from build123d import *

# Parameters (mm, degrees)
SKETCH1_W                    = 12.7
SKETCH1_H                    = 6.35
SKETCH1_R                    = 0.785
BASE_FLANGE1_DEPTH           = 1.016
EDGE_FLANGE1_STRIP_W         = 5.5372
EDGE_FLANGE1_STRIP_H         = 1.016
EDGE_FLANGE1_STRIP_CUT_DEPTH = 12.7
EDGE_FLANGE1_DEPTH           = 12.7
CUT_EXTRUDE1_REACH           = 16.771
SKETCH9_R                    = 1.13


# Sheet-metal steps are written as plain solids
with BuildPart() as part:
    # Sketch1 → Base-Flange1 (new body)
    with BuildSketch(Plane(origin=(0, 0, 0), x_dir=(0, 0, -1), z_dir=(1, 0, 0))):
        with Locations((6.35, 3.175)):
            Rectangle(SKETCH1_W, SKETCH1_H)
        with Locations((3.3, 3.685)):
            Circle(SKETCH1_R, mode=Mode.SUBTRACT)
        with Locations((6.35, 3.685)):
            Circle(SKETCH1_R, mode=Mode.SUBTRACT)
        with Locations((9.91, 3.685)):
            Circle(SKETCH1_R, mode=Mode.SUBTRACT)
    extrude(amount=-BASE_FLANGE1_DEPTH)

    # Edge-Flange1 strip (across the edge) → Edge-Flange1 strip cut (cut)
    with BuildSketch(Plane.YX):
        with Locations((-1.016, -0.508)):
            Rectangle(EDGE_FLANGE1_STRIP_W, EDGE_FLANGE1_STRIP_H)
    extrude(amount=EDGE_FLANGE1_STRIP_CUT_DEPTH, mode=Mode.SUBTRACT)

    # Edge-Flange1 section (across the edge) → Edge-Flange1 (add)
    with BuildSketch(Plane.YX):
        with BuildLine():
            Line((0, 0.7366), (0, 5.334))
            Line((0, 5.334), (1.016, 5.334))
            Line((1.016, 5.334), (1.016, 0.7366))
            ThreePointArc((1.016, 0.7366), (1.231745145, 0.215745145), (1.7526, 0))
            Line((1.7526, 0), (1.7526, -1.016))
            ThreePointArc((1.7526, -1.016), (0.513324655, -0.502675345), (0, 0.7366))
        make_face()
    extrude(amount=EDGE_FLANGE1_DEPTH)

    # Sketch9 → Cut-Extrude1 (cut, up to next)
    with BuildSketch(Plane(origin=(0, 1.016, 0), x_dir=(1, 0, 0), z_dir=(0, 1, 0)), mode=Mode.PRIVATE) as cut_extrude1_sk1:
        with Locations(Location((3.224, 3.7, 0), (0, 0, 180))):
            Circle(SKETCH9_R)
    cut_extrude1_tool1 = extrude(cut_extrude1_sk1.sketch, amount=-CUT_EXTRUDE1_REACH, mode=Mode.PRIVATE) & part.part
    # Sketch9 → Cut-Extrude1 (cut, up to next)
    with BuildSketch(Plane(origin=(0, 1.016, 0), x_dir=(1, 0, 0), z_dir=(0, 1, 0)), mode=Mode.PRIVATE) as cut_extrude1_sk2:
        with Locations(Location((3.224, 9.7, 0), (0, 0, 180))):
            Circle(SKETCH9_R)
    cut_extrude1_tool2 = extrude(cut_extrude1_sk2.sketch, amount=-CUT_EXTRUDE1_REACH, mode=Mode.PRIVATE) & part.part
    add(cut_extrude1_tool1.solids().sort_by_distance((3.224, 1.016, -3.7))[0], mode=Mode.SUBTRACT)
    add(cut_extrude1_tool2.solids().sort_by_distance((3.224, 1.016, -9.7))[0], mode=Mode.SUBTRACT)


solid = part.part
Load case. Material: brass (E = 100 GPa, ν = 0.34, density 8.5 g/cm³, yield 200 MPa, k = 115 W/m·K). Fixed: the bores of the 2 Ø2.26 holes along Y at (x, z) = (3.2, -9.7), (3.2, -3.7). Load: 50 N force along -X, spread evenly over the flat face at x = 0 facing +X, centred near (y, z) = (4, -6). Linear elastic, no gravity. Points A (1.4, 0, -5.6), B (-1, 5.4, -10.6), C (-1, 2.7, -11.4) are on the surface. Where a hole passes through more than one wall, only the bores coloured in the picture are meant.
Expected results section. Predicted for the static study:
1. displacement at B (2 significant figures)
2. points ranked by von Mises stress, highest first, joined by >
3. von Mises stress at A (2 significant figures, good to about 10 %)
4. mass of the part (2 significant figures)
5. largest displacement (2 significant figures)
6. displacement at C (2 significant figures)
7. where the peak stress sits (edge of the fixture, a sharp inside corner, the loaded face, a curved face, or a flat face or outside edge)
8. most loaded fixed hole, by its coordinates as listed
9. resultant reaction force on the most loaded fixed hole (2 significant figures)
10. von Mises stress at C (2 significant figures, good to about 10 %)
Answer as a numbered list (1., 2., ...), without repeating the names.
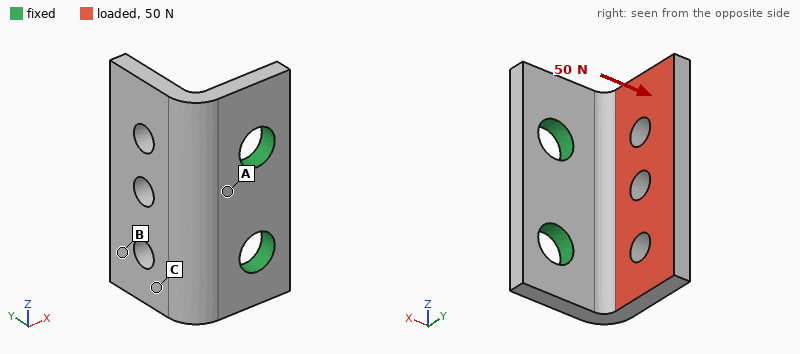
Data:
1. 31 µm
2. A > C > B
3. 66 MPa
4. 1.1 g
5. 38 µm
6. 15 µm
7. a flat face or outside edge
8. (3.2, -3.7)
9. 27 N
10. 39 MPa
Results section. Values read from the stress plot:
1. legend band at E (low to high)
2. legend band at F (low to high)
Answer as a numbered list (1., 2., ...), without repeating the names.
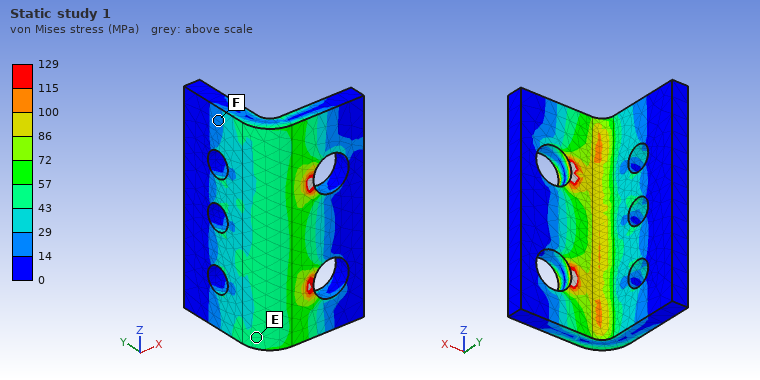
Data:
1. 43 to 57 MPa
2. 14 to 29 MPa
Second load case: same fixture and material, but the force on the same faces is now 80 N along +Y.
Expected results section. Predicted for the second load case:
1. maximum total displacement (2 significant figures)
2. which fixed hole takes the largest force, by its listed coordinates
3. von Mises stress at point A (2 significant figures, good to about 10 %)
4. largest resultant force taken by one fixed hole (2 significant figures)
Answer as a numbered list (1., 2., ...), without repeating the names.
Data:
1. 12 µm
2. (3.2, -3.7)
3. 39 MPa
4. 44 N
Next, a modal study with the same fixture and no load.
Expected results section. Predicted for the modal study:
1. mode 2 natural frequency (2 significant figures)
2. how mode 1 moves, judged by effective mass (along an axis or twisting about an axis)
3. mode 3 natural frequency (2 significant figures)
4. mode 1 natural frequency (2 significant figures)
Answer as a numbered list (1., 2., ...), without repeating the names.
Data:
1. 15 kHz
2. along X
3. 25 kHz
4. 9800 Hz
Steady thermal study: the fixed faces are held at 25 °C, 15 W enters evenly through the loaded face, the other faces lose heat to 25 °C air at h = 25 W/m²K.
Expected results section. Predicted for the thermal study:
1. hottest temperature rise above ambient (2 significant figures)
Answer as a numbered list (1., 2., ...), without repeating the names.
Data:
1. 71 K
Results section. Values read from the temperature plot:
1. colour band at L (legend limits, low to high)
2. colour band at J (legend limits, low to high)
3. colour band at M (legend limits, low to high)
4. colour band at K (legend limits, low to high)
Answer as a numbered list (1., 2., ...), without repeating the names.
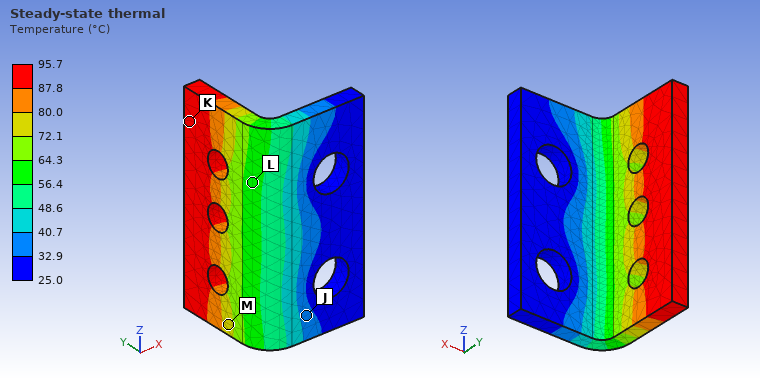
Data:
1. 56.4 to 64.3 °C
2. 32.9 to 40.7 °C
3. 72.1 to 80.0 °C
4. 87.8 to 95.7 °C
